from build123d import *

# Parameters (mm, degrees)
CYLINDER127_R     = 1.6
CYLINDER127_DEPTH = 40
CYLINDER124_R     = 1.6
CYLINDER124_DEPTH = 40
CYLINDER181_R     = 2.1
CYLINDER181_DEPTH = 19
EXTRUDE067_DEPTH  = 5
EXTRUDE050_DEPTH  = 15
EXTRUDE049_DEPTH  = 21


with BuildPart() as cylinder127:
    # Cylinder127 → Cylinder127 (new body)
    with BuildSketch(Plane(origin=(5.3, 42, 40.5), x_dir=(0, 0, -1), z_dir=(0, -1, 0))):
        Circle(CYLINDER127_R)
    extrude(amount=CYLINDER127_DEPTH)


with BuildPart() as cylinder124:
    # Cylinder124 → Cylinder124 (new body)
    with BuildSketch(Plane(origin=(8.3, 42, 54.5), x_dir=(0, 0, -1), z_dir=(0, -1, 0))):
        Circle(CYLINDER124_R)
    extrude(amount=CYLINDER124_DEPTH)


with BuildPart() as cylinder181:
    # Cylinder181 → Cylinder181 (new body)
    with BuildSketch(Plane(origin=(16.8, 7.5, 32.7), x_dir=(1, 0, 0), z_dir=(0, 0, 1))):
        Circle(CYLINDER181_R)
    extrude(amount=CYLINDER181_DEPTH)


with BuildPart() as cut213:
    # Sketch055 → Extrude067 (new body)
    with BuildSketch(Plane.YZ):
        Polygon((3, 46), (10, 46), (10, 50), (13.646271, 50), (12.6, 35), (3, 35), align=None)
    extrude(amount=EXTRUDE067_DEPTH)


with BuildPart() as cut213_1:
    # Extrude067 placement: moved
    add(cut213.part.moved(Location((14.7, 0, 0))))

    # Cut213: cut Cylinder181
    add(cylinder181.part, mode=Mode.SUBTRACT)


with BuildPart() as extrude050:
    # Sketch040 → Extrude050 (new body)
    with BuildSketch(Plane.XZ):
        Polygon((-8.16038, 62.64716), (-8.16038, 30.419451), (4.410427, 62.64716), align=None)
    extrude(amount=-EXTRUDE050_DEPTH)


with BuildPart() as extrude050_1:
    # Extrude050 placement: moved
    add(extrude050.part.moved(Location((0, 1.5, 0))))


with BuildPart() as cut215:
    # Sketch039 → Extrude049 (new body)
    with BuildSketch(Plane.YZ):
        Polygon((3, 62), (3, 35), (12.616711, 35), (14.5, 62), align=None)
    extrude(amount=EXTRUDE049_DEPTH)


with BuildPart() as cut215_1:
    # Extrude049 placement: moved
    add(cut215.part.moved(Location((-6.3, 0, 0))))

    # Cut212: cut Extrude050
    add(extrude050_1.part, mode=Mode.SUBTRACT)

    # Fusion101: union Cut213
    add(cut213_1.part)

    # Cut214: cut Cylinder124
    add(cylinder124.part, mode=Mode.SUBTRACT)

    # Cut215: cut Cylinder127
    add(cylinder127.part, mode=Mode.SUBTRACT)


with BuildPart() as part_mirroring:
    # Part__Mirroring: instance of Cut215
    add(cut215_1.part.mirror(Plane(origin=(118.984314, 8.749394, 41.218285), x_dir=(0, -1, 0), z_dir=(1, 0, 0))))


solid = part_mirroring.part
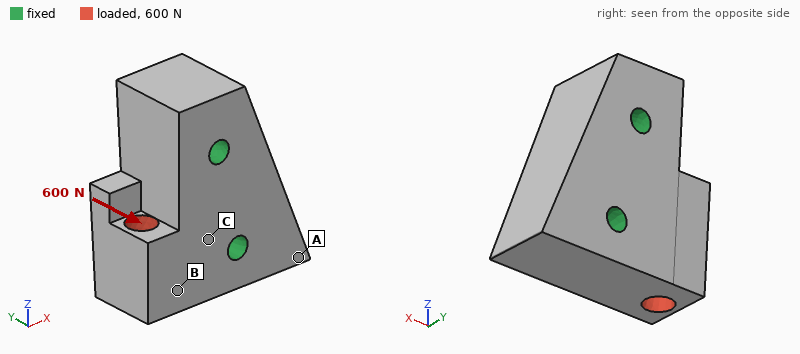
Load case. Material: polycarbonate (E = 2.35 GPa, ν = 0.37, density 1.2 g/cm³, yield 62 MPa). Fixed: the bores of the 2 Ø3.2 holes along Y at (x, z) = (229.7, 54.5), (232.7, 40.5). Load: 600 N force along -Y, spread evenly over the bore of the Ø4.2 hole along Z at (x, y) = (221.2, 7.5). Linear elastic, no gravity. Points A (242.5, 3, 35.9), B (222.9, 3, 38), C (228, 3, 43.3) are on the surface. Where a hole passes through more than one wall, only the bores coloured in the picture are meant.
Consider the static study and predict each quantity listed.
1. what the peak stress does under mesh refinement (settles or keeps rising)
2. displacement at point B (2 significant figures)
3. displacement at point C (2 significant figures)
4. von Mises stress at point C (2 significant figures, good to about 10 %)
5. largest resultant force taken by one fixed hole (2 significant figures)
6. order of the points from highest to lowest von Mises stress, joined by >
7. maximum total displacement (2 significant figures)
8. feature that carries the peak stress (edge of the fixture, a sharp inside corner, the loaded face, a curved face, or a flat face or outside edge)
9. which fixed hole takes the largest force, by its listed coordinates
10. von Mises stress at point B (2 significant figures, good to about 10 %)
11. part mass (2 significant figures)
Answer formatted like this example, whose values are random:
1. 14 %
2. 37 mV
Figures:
1. keeps rising
2. 0.17 mm
3. 0.063 mm
4. 15 MPa
5. 450 N
6. C > B > A
7. 0.29 mm
8. edge of the fixture
9. (232.7, 40.5)
10. 11 MPa
11. 5.7 g
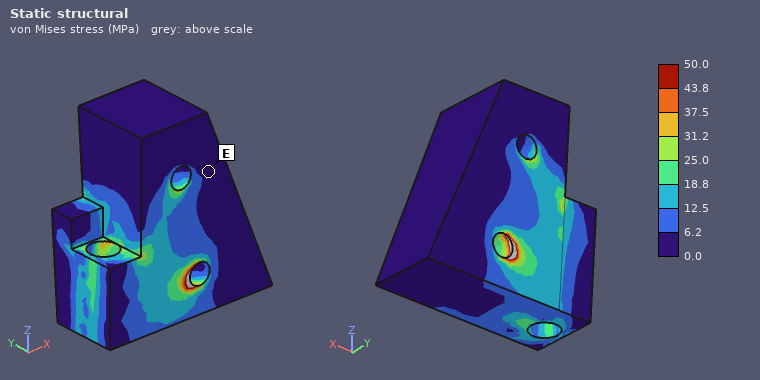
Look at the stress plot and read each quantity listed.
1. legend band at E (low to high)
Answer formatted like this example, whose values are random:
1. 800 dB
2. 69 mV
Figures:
1. 0.0 to 6.2 MPa
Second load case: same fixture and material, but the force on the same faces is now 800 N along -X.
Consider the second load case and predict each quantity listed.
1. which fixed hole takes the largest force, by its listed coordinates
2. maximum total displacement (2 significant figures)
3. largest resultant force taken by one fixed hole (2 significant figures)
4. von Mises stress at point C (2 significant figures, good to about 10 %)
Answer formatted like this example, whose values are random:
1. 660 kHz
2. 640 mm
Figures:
1. (232.7, 40.5)
2. 0.11 mm
3. 770 N
4. 8.2 MPa
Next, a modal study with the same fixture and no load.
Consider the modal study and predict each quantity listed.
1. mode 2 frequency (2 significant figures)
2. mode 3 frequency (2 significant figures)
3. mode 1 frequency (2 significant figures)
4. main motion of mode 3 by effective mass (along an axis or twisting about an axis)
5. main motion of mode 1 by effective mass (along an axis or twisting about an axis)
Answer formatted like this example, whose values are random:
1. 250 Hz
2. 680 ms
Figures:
1. 14 kHz
2. 15 kHz
3. 9800 Hz
4. along Y
5. along Y
